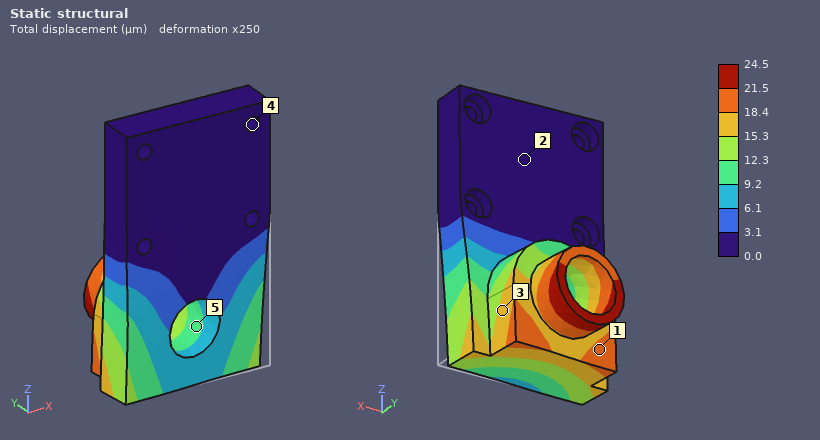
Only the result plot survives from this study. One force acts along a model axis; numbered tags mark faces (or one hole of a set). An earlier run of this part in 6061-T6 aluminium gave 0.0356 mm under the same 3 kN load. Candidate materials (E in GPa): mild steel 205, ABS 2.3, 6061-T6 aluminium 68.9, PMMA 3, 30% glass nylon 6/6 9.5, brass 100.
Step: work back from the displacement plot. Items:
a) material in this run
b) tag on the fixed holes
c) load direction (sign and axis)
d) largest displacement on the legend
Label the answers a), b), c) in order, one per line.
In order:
a) brass
b) 4
c) -X
d) 24.5 µm
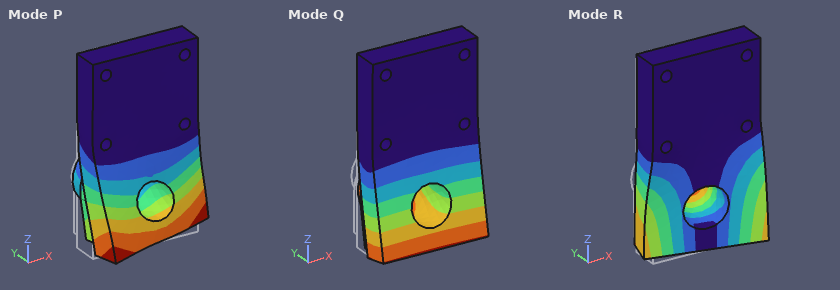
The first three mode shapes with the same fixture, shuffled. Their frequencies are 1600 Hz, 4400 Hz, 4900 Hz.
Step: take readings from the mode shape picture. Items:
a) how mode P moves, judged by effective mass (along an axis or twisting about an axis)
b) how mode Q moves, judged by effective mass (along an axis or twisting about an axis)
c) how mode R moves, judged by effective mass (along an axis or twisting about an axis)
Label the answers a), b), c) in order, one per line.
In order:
a) along X
b) along Y
c) along X
